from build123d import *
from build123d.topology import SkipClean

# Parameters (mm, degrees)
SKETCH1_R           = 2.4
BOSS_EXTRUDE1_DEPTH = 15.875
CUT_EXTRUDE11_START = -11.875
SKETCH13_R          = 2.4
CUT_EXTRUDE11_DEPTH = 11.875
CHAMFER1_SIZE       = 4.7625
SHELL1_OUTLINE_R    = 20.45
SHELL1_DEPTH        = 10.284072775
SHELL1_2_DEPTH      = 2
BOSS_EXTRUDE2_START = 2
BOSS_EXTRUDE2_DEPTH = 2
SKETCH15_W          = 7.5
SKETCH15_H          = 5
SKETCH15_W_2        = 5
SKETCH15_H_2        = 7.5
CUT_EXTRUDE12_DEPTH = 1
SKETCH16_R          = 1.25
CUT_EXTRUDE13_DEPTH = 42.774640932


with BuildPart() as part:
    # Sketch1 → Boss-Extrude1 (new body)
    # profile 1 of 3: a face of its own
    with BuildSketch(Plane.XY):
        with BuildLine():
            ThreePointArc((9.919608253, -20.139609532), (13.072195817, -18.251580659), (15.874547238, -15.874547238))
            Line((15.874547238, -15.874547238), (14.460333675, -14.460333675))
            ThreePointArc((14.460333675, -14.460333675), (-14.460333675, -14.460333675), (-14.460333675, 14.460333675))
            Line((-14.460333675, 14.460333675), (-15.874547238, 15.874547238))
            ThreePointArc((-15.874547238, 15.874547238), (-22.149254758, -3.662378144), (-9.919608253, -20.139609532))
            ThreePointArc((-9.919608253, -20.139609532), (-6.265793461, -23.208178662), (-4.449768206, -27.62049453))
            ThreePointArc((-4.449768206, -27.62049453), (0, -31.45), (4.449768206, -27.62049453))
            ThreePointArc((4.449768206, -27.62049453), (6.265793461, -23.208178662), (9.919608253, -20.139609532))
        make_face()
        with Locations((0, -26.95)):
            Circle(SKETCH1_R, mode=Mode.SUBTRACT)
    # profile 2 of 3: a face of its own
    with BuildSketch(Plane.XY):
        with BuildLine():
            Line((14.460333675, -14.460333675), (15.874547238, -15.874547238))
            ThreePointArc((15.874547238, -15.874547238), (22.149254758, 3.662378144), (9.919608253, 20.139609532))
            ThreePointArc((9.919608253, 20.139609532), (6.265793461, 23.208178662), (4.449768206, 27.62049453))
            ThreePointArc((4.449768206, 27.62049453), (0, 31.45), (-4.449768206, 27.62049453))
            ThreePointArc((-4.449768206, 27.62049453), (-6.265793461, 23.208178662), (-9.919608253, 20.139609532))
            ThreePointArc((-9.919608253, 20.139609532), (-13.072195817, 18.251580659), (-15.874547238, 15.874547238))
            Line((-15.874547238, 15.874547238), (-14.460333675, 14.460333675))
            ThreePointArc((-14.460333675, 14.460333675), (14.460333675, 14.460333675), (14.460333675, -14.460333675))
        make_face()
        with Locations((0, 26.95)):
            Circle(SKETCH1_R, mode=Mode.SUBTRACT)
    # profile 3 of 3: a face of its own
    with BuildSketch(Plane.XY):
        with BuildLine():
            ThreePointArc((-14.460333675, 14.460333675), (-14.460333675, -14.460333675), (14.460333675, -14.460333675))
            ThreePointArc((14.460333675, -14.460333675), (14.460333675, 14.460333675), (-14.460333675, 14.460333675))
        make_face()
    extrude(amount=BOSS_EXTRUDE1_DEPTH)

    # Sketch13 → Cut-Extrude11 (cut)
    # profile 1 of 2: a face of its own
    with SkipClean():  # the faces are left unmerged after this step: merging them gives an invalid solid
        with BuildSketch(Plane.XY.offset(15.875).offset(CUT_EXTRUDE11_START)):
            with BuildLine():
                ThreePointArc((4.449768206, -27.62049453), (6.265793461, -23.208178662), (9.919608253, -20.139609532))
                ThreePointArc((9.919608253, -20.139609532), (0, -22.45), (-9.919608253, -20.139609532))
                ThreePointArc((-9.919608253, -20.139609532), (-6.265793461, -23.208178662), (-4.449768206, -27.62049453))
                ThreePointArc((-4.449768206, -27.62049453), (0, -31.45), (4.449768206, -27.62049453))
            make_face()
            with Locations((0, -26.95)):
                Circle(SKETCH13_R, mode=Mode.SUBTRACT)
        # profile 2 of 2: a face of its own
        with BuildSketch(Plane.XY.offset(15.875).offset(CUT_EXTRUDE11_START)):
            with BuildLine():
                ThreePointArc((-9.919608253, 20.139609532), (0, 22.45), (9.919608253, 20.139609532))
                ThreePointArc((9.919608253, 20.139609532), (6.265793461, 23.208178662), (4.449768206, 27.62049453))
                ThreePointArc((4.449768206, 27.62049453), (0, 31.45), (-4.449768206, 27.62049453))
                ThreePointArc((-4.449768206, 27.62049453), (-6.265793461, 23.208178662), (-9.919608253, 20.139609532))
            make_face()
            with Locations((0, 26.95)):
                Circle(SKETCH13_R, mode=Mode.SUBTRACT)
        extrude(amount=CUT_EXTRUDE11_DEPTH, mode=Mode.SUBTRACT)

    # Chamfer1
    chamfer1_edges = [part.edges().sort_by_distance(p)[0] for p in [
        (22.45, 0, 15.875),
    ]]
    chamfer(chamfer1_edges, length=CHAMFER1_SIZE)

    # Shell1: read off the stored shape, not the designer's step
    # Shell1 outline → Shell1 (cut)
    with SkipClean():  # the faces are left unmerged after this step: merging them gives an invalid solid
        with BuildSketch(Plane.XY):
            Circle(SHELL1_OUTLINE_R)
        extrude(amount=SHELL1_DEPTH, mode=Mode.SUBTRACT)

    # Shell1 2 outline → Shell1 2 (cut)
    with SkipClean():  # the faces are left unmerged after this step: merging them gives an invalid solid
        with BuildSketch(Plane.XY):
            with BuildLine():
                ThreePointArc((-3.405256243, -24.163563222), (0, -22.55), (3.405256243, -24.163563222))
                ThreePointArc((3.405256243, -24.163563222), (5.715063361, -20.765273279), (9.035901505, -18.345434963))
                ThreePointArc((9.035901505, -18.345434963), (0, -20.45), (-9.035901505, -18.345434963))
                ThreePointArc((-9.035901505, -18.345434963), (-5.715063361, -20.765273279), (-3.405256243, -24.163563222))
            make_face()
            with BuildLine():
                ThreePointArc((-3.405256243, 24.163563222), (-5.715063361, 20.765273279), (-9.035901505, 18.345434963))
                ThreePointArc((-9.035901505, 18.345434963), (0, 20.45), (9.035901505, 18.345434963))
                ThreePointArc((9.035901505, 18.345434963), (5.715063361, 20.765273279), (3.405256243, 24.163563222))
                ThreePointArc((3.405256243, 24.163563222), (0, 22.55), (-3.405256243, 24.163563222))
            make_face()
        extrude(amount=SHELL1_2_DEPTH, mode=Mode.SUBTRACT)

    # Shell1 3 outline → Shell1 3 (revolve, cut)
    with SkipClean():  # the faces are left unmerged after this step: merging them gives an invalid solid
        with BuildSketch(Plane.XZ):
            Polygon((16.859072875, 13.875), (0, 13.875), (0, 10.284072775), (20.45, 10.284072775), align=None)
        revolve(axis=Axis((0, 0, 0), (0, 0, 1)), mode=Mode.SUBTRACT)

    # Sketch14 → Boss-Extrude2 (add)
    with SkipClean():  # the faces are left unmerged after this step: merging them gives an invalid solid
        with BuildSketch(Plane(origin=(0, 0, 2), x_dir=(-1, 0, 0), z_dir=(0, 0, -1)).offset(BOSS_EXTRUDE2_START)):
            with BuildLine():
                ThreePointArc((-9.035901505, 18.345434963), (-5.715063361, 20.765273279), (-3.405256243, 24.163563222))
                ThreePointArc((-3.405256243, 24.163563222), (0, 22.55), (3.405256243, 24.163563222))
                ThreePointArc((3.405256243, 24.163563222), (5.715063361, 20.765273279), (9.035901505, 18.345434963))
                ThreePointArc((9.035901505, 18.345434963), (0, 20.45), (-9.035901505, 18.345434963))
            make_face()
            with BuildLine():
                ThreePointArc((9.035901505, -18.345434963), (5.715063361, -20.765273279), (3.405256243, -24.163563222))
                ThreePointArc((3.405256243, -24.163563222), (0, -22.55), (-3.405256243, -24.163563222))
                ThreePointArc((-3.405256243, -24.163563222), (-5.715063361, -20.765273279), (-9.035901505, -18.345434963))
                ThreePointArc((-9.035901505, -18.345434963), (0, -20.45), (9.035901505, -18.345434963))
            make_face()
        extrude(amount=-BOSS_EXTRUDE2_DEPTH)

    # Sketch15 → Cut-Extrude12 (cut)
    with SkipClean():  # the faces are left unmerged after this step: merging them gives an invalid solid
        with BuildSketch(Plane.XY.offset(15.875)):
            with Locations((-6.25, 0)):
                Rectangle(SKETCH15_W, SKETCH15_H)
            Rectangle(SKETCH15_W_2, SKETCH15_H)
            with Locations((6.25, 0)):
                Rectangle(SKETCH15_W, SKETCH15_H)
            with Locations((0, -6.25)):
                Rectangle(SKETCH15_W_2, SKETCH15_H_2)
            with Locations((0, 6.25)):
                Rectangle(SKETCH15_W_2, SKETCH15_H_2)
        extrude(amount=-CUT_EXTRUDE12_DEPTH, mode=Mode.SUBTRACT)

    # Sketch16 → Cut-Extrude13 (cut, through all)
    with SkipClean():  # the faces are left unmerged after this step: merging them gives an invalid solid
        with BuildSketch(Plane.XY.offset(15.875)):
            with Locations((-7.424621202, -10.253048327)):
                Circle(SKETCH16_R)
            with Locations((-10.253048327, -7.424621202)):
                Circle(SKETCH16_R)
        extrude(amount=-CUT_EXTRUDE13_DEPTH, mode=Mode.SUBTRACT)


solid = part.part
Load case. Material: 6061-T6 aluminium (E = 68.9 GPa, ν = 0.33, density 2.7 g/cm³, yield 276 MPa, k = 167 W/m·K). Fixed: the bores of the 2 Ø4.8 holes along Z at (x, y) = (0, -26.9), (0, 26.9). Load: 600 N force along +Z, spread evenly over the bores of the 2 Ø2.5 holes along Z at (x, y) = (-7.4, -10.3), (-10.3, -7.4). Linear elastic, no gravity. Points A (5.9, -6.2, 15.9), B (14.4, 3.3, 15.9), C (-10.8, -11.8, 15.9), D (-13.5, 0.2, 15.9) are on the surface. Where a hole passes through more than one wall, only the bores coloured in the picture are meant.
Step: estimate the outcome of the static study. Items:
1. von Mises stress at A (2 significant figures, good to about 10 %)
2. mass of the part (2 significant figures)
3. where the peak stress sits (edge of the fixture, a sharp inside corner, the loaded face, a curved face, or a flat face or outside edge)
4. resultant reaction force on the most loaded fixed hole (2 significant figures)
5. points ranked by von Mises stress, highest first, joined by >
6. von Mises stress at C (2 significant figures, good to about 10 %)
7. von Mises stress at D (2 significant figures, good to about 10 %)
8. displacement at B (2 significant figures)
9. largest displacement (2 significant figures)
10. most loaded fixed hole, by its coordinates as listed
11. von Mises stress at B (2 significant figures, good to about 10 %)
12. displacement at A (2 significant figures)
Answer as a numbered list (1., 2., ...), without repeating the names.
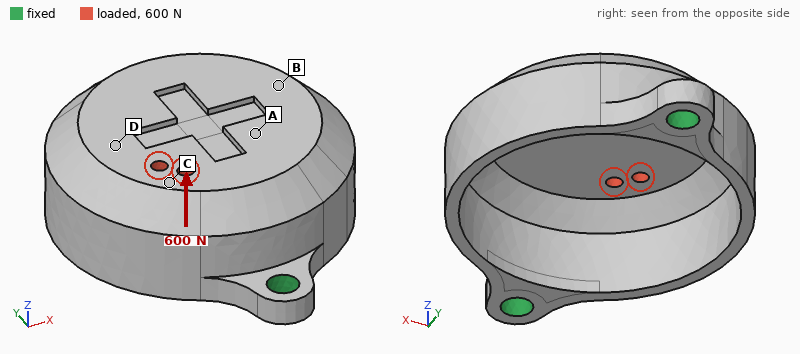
1. 24 MPa
2. 18 g
3. the loaded face
4. 460 N
5. C > D > A > B
6. 90 MPa
7. 40 MPa
8. 36 µm
9. 88 µm
10. (0, -26.9)
11. 12 MPa
12. 35 µm
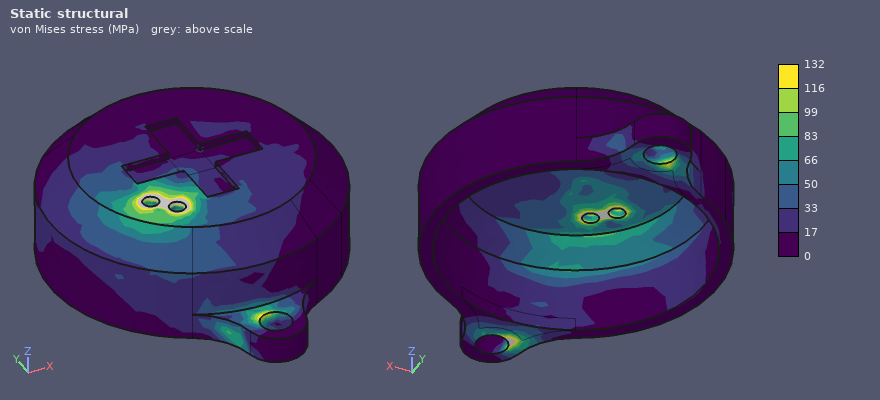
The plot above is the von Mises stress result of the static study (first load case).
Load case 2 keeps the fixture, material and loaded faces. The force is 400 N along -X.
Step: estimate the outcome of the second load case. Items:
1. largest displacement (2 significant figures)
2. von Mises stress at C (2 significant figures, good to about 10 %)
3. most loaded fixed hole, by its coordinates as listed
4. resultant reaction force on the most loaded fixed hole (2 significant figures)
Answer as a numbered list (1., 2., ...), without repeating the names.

1. 54 µm
2. 11 MPa
3. (0, -26.9)
4. 270 N
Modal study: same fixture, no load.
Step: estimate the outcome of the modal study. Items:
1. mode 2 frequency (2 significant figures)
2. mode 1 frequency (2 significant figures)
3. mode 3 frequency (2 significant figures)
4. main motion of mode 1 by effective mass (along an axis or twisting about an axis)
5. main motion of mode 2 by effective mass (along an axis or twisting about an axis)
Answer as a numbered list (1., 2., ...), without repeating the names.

1. 7100 Hz
2. 3700 Hz
3. 8000 Hz
4. along X
5. along Y
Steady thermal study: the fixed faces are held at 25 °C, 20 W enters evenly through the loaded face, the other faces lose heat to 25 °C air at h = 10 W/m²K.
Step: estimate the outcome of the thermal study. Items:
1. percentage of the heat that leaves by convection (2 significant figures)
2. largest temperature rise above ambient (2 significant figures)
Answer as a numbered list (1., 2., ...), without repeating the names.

1. 5.7 %
2. 45 K
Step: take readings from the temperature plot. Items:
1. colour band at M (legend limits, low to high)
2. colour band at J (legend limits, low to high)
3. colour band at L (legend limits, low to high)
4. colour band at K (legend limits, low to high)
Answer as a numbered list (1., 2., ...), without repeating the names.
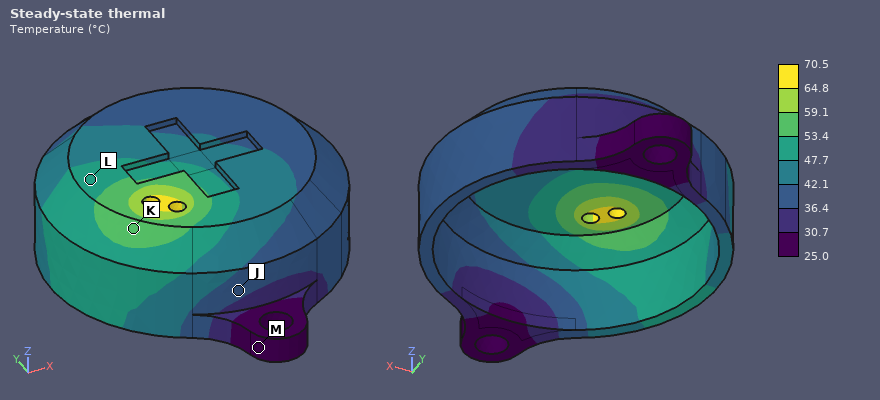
1. 25.0 to 30.7 °C
2. 36.4 to 42.1 °C
3. 47.7 to 53.4 °C
4. 53.4 to 59.1 °C
